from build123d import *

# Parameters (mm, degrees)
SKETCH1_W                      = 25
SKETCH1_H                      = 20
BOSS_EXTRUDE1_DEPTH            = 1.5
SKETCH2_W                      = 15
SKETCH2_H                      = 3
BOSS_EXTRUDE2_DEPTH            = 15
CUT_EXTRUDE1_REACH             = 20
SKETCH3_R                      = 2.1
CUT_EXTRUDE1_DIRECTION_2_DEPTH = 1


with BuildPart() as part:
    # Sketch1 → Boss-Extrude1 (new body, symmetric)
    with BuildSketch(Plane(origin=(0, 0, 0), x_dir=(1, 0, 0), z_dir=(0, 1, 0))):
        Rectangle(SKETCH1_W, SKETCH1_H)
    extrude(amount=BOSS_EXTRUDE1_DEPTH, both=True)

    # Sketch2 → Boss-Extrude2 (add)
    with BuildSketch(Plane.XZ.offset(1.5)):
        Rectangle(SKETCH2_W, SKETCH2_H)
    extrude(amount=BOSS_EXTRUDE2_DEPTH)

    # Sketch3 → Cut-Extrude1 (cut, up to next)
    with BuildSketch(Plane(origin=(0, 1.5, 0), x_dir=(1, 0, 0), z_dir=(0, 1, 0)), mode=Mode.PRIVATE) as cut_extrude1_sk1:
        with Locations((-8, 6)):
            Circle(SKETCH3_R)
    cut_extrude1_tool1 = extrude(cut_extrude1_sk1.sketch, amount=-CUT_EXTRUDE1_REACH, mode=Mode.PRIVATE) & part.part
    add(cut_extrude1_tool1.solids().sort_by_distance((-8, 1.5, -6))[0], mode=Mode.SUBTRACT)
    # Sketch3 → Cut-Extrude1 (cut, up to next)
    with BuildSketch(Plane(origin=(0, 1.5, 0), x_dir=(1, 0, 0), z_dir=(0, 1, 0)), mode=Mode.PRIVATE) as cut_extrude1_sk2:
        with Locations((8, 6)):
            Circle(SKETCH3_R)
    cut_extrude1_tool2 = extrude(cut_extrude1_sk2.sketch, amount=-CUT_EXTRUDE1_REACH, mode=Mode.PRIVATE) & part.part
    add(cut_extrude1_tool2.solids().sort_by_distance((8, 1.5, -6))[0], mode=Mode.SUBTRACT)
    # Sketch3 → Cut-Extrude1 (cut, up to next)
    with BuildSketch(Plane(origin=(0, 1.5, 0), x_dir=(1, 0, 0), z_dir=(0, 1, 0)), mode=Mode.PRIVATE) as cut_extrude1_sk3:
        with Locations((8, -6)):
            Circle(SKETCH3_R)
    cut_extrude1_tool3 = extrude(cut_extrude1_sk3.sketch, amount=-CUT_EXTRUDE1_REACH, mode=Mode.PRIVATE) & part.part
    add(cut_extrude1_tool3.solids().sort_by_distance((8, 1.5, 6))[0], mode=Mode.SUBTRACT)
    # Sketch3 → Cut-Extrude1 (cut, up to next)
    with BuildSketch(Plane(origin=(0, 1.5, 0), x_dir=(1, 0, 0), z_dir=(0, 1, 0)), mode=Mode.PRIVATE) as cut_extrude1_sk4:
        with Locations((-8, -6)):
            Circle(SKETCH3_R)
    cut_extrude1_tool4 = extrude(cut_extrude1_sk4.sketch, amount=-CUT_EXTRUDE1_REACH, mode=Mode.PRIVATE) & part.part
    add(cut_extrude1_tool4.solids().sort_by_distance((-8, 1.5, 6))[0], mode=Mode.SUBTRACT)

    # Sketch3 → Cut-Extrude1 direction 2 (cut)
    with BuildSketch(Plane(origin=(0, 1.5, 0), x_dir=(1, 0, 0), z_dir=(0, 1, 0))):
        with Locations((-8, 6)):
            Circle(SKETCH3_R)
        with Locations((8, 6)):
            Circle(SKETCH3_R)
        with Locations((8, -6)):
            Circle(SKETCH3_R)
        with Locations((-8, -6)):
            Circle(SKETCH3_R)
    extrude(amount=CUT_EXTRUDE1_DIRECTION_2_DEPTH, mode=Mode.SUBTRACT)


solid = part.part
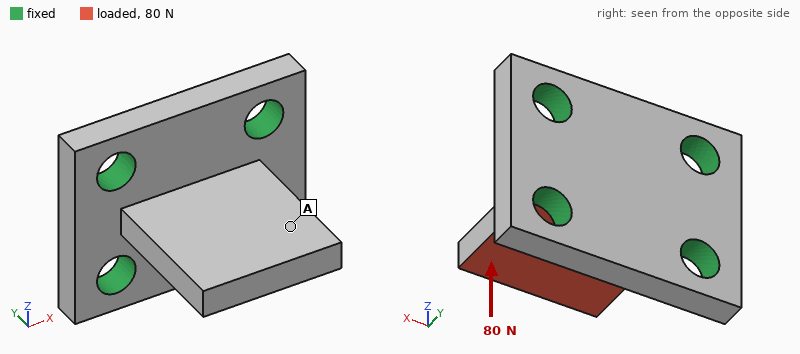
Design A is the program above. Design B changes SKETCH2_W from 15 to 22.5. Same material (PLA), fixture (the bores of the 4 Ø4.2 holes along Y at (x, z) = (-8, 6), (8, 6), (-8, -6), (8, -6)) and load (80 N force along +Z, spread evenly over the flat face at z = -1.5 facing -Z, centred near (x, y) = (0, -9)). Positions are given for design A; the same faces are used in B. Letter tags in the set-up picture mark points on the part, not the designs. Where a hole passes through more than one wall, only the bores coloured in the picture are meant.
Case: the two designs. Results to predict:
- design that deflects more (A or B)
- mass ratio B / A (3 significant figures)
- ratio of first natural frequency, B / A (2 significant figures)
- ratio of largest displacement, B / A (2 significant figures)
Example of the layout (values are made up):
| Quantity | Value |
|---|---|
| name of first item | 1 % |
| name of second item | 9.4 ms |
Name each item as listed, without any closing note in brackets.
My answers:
| Quantity | Value |
|---|---|
| design that deflects more | A |
| mass ratio B / A | 1.17 |
| ratio of first natural frequency, B / A | 1.0 |
| ratio of largest displacement, B / A | 0.66 |
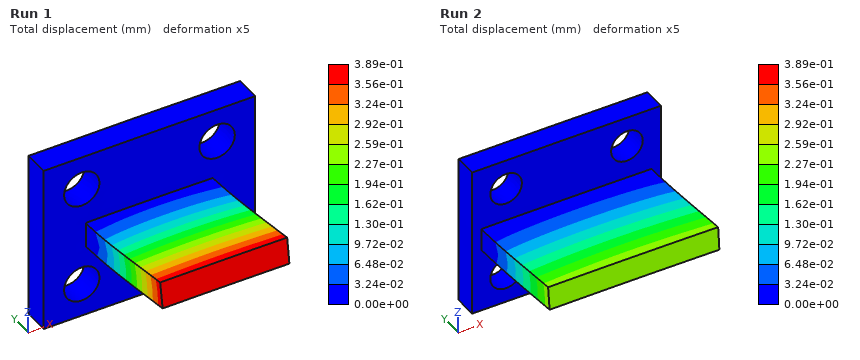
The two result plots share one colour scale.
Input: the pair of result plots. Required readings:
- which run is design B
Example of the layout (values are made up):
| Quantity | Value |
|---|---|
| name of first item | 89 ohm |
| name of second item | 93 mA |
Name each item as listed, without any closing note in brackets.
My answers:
| Quantity | Value |
|---|---|
| which run is design B | Run 2 |
